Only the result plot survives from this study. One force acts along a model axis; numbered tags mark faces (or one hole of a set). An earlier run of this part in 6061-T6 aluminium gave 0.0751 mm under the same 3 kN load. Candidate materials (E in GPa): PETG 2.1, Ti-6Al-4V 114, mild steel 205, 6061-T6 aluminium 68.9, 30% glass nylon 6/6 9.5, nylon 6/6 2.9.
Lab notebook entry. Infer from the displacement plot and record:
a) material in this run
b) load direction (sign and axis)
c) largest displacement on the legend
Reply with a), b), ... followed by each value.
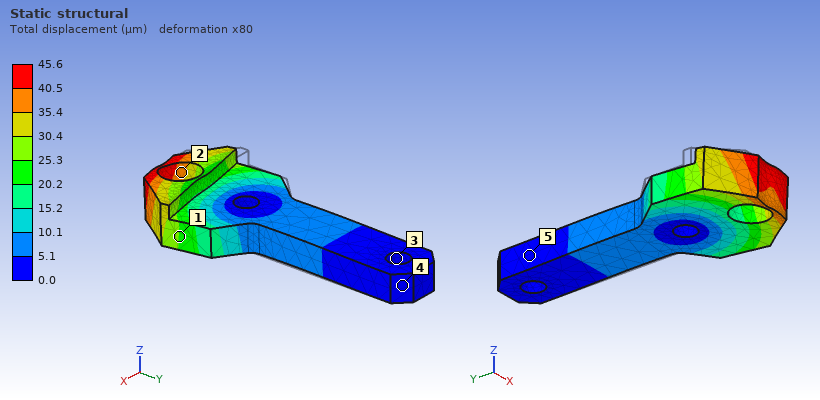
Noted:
a) Ti-6Al-4V
b) +X
c) 45.6 µm
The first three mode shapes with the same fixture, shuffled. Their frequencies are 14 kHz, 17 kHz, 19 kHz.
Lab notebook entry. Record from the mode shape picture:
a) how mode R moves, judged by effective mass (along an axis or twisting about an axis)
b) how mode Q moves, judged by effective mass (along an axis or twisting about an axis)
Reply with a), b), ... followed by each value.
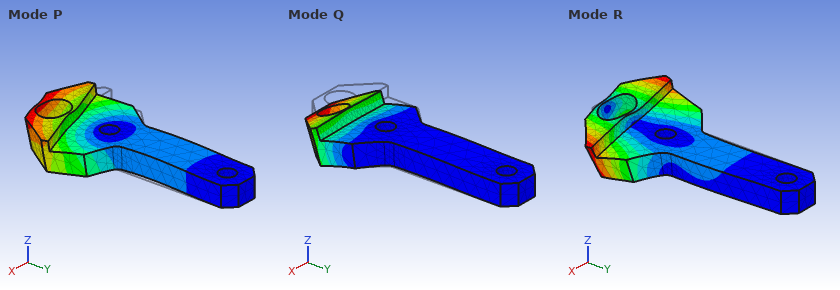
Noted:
a) twisting about Y
b) along Z
